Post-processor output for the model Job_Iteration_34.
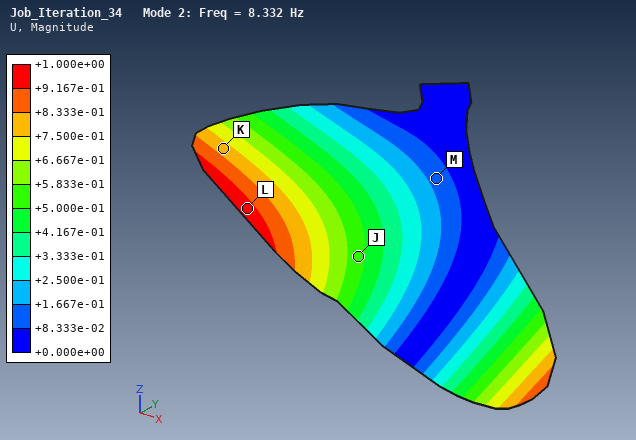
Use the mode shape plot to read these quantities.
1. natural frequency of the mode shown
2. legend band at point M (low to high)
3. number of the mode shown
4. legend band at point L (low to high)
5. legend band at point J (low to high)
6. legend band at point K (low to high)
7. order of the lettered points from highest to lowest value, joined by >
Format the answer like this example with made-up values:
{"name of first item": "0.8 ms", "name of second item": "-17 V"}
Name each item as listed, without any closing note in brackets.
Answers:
{"natural frequency of the mode shown": "8.332 Hz", "legend band at point M": "+8.333e-02 to +1.667e-01", "number of the mode shown": "2", "legend band at point L": "+9.167e-01 to +1.000e+00", "legend band at point J": "+5.000e-01 to +5.833e-01", "legend band at point K": "+7.500e-01 to +8.333e-01", "order of the lettered points from highest to lowest value, joined by >": "L > K > J > M"}
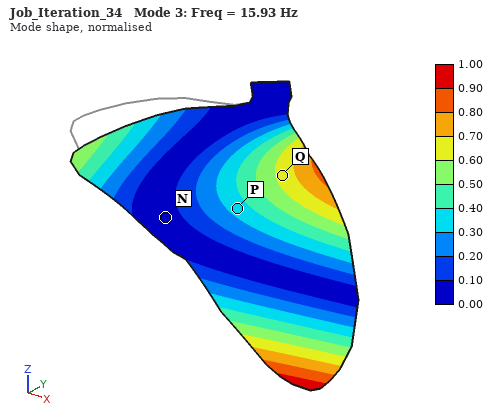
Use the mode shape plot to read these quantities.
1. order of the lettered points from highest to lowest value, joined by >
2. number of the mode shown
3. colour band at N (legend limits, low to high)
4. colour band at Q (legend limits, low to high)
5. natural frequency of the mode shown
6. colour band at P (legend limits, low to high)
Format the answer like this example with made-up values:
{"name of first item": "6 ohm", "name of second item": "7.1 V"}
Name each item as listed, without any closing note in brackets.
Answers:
{"order of the lettered points from highest to lowest value, joined by >": "Q > P > N", "number of the mode shown": "3", "colour band at N": "0.00 to 0.10", "colour band at Q": "0.60 to 0.70", "natural frequency of the mode shown": "15.93 Hz", "colour band at P": "0.30 to 0.40"}
